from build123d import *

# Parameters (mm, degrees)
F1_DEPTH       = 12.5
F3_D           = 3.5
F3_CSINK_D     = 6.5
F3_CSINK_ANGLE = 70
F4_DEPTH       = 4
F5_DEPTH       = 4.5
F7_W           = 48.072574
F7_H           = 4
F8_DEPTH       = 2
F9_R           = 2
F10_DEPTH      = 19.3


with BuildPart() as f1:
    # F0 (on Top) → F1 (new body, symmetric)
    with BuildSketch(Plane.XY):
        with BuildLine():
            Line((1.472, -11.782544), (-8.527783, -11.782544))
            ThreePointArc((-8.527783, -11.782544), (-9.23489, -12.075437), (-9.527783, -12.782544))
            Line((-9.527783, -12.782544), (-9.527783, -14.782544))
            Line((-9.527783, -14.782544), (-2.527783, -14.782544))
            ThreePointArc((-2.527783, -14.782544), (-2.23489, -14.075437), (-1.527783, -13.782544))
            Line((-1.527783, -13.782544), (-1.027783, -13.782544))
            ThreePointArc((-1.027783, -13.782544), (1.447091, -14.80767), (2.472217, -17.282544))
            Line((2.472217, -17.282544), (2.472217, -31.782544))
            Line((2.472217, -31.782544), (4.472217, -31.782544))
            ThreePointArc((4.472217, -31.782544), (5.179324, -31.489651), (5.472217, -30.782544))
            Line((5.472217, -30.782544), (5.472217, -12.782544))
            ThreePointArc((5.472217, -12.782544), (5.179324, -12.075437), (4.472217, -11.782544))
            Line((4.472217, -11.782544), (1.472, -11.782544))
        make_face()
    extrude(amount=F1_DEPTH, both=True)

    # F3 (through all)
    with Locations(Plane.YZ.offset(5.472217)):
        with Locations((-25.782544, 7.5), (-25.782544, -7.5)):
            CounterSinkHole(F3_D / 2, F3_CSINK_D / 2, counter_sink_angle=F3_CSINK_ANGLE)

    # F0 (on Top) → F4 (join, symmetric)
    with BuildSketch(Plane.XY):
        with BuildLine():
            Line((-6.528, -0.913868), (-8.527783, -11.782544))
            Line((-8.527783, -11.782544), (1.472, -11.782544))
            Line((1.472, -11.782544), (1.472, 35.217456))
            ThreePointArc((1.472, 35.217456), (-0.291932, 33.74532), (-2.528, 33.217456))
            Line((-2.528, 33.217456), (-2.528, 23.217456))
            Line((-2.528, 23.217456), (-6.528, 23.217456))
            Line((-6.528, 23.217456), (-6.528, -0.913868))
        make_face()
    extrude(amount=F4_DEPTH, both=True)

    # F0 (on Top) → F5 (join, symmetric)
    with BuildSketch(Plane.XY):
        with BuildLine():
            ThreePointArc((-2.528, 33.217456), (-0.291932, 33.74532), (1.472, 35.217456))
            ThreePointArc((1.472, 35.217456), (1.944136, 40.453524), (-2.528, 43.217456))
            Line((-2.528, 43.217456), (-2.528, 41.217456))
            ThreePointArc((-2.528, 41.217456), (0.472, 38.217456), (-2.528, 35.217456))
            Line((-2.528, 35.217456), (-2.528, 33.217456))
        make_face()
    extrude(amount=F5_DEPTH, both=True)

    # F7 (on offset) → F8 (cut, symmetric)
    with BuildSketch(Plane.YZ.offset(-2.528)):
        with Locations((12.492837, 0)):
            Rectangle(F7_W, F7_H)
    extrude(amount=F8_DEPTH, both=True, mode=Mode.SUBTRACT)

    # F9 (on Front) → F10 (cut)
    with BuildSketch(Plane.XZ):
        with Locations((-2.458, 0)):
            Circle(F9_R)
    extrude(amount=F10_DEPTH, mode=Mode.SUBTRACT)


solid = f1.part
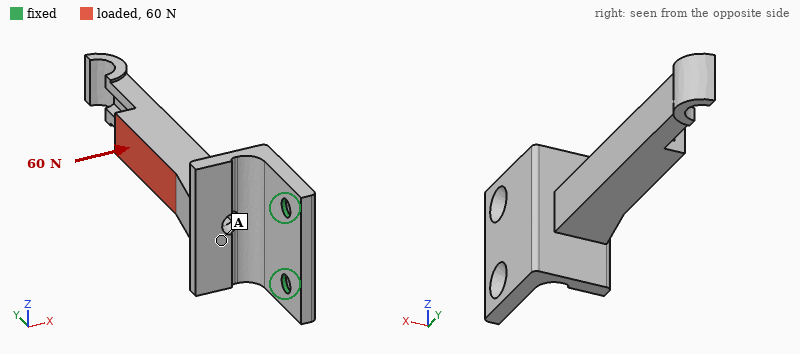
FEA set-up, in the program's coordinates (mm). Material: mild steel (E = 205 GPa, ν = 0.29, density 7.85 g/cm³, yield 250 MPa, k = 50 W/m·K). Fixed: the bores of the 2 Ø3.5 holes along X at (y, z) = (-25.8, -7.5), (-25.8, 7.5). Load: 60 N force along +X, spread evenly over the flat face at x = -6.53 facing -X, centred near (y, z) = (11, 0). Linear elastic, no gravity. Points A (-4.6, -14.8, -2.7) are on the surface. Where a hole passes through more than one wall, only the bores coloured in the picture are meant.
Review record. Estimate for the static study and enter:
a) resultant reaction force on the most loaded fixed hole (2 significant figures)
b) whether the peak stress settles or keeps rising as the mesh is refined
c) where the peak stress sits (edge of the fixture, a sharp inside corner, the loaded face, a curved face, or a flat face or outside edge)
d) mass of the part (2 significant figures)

41 N
keeps rising
edge of the fixture
35 g
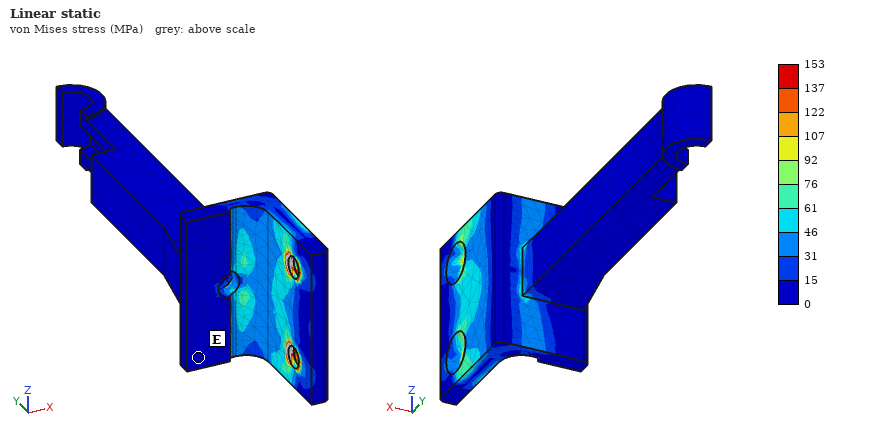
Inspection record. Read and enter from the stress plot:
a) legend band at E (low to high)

0 to 15 MPa
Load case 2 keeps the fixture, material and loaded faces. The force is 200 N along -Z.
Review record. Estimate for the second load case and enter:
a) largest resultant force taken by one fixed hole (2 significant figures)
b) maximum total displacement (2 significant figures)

450 N
95 µm
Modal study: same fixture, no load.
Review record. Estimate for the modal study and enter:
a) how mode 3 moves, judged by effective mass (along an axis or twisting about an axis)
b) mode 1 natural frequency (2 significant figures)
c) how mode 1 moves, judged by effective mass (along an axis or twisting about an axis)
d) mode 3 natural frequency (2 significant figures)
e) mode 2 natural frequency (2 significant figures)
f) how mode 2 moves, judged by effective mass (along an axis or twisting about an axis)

along X
750 Hz
along X
5200 Hz
2200 Hz
along Z
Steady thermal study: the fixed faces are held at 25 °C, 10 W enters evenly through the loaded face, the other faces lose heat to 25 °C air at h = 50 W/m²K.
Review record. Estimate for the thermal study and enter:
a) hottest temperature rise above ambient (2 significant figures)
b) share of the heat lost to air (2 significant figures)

70 K
63 %
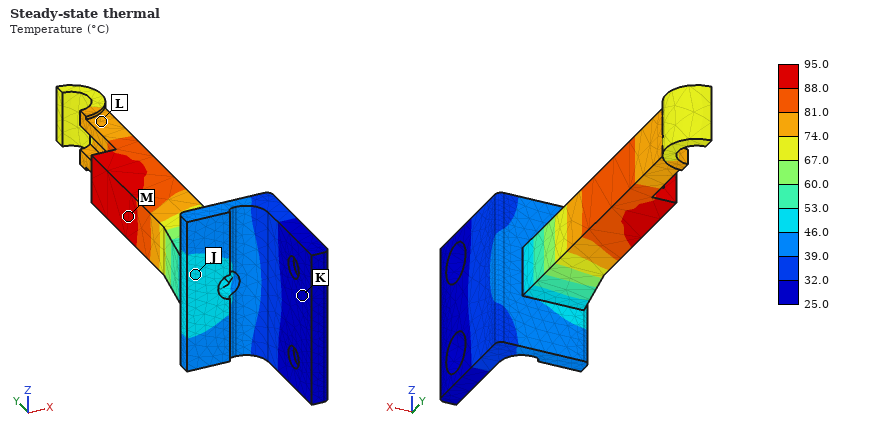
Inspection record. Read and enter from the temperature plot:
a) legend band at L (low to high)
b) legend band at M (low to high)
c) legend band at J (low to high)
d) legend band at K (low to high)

74.0 to 81.0 °C
88.0 to 95.0 °C
46.0 to 53.0 °C
25.0 to 32.0 °C
